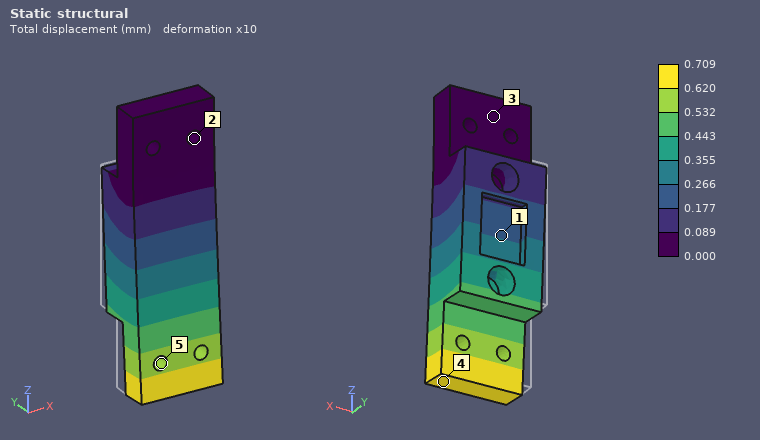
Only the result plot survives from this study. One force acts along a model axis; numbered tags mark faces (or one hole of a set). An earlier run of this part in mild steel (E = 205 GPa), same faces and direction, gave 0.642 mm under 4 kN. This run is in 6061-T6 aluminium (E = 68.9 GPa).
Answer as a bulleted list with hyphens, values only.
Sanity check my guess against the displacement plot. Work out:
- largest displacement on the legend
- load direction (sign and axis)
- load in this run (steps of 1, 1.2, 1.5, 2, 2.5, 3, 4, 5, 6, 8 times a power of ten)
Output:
- 0.709 mm
- -Y
- 1.5 kN
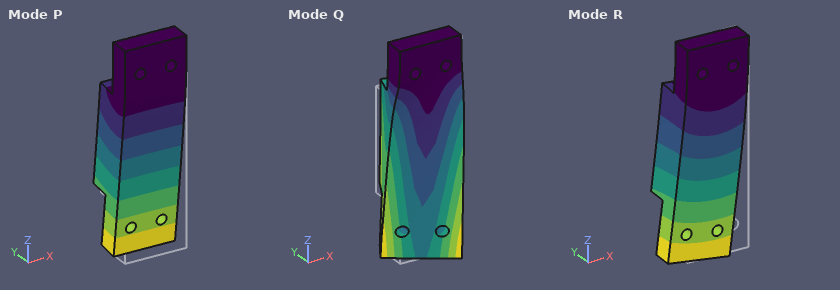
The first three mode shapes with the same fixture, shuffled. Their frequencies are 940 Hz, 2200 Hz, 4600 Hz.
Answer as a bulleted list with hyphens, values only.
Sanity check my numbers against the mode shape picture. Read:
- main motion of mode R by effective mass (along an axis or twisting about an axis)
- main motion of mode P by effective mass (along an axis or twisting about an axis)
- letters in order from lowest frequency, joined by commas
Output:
- along X
- along Y
- P, R, Q
